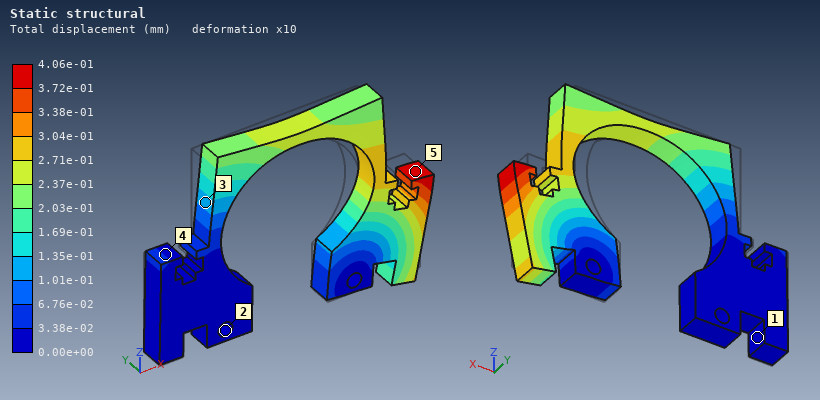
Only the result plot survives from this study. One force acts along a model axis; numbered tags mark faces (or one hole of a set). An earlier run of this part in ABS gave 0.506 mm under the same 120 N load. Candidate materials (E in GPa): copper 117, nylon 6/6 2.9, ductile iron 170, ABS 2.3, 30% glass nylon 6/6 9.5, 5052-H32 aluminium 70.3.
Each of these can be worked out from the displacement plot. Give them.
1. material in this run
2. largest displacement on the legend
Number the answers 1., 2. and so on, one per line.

1. nylon 6/6
2. 4.06e-01 mm
